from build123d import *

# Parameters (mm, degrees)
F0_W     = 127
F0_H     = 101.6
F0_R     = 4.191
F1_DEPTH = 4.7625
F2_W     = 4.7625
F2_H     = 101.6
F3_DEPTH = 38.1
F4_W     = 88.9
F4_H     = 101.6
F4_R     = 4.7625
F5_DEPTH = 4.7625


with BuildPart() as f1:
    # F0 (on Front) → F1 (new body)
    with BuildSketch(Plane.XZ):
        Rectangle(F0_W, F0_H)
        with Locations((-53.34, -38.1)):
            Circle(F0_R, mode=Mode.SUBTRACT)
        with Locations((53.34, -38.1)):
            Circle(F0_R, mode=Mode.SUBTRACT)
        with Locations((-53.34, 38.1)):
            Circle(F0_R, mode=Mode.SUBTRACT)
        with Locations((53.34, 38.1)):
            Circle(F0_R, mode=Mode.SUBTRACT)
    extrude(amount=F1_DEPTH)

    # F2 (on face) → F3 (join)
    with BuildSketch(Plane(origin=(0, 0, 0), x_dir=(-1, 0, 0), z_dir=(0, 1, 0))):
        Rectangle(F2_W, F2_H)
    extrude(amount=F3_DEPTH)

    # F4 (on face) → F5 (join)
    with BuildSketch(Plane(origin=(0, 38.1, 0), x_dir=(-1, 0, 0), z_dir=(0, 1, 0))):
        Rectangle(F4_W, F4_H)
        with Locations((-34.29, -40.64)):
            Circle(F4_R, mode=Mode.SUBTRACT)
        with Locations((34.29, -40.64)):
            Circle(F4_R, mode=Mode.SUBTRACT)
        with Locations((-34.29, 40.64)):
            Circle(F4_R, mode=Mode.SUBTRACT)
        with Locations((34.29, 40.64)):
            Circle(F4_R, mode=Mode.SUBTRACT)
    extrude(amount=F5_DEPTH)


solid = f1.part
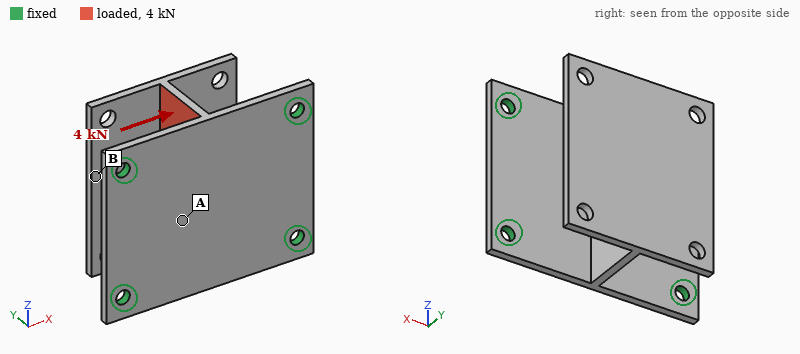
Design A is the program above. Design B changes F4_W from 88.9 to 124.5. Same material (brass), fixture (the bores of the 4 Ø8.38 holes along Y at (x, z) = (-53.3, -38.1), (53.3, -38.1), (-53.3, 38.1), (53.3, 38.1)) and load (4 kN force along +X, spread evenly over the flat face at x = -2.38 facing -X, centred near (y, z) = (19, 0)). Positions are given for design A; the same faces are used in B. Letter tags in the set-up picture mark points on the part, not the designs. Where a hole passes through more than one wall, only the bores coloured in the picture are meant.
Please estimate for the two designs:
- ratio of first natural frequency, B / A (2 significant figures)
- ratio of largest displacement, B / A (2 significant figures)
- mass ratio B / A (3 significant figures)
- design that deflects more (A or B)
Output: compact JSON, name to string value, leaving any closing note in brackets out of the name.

{"ratio of first natural frequency, B / A": "0.70", "ratio of largest displacement, B / A": "1.2", "mass ratio B / A": "1.14", "design that deflects more": "B"}
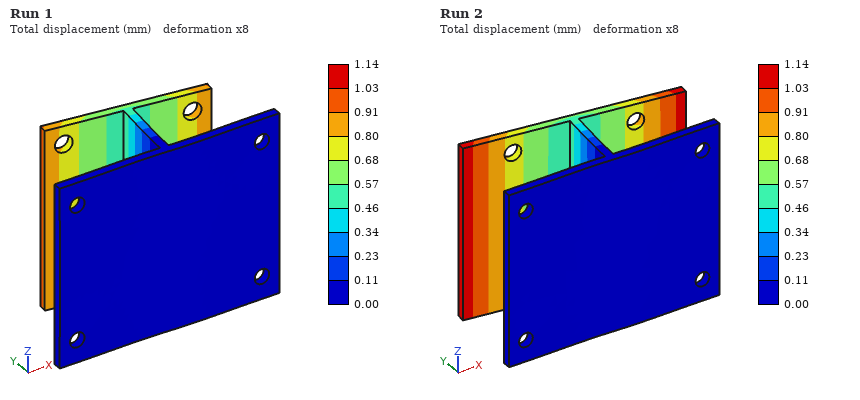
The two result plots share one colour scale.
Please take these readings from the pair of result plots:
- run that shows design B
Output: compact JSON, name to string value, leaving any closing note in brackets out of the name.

{"run that shows design B": "Run 2"}
